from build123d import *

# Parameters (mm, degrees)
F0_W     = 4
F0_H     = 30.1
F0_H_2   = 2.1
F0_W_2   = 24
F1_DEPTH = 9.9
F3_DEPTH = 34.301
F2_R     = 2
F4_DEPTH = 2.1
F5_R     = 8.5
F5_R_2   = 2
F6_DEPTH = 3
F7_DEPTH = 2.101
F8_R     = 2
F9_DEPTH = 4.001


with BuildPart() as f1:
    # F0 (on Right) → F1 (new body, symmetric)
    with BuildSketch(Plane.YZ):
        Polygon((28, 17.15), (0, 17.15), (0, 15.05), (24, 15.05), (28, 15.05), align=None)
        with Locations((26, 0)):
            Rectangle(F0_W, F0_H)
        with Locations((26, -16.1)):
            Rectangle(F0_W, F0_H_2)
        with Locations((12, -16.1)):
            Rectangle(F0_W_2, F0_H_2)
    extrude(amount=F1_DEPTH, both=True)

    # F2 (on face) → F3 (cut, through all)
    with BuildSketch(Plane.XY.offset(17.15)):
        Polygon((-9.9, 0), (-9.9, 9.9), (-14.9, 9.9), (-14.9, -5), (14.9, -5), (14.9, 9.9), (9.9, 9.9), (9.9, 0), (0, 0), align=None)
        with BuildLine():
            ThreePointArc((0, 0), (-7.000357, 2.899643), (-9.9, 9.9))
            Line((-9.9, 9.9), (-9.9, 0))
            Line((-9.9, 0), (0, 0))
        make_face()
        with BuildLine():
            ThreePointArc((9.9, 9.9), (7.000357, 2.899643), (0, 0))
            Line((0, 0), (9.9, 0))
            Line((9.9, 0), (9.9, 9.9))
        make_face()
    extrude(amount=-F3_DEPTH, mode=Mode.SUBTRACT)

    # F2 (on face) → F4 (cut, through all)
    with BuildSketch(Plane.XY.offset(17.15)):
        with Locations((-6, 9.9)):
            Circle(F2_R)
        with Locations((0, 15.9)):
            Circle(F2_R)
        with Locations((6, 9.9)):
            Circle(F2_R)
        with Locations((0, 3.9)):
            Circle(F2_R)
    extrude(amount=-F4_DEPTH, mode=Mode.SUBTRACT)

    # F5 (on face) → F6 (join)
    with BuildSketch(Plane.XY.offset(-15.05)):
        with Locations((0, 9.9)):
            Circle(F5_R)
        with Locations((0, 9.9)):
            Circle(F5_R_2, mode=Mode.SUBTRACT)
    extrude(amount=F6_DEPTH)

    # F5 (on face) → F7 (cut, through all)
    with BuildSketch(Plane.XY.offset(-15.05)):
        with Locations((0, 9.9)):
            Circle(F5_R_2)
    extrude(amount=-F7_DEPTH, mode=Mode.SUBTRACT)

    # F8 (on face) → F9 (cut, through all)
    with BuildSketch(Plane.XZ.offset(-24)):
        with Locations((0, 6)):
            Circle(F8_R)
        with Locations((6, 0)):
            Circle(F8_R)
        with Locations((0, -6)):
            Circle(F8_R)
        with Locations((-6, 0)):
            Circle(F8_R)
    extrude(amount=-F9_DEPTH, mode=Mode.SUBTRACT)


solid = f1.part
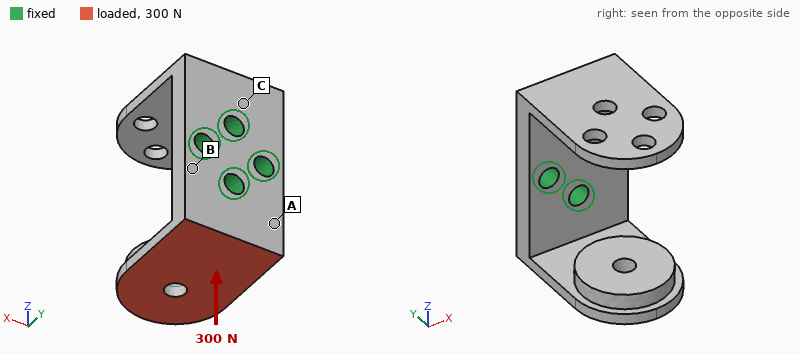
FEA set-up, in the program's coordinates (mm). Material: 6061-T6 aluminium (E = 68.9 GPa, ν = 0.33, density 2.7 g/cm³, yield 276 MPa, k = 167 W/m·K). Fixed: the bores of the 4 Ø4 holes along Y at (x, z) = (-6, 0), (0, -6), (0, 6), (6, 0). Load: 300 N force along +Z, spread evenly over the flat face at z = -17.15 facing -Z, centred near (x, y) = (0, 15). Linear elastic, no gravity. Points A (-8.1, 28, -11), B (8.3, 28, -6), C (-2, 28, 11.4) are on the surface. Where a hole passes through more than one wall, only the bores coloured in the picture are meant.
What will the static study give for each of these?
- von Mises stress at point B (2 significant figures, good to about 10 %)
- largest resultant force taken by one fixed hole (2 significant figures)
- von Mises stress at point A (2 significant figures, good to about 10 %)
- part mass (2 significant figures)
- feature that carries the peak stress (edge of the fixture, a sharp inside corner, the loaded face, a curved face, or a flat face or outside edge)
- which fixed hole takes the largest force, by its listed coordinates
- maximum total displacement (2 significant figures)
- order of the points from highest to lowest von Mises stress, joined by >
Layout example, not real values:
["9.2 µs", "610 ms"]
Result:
["27 MPa", "280 N", "51 MPa", "13 g", "the loaded face", "(0, -6)", "0.43 mm", "A > B > C"]
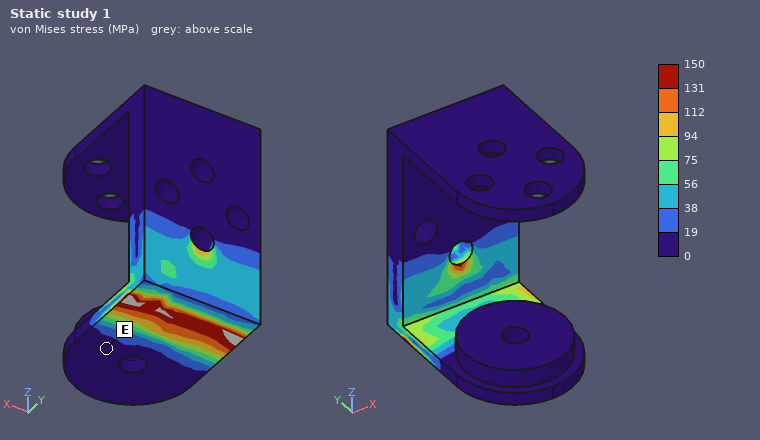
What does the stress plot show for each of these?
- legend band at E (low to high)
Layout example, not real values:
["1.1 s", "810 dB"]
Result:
["0 to 19 MPa"]
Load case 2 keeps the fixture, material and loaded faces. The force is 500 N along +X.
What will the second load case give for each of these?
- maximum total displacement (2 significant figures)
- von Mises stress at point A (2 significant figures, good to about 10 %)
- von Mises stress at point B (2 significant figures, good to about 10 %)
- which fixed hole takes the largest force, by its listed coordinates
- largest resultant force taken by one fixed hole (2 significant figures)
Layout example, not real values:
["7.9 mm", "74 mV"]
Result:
["0.13 mm", "47 MPa", "65 MPa", "(0, -6)", "560 N"]
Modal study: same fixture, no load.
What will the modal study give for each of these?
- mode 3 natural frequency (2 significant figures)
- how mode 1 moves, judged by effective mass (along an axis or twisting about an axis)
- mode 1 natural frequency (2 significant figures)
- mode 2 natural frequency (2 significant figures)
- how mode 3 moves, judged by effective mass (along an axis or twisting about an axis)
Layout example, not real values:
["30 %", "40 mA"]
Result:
["4800 Hz", "along Z", "2300 Hz", "3100 Hz", "along X"]
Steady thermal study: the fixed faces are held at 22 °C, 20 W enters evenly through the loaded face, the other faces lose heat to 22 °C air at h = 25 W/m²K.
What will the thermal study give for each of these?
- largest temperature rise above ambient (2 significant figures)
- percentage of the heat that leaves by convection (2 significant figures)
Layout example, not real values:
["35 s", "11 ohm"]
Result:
["38 K", "3.7 %"]
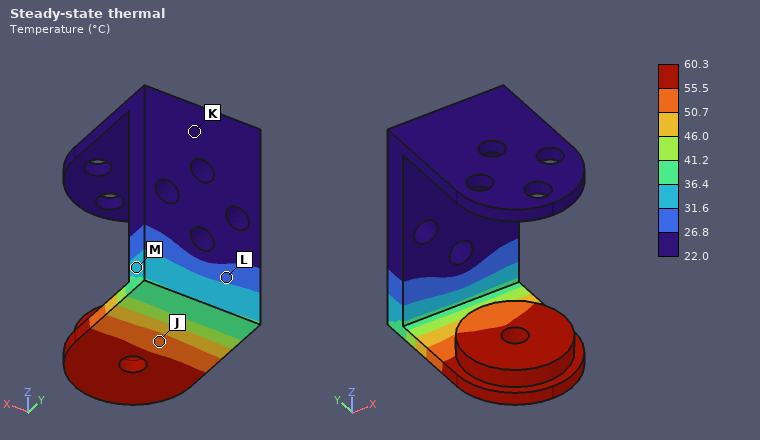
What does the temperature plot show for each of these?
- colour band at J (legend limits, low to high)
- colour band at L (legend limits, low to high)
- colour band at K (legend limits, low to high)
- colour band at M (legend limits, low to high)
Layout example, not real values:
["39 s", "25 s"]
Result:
["50.7 to 55.5 °C", "26.8 to 31.6 °C", "22.0 to 26.8 °C", "31.6 to 36.4 °C"]
